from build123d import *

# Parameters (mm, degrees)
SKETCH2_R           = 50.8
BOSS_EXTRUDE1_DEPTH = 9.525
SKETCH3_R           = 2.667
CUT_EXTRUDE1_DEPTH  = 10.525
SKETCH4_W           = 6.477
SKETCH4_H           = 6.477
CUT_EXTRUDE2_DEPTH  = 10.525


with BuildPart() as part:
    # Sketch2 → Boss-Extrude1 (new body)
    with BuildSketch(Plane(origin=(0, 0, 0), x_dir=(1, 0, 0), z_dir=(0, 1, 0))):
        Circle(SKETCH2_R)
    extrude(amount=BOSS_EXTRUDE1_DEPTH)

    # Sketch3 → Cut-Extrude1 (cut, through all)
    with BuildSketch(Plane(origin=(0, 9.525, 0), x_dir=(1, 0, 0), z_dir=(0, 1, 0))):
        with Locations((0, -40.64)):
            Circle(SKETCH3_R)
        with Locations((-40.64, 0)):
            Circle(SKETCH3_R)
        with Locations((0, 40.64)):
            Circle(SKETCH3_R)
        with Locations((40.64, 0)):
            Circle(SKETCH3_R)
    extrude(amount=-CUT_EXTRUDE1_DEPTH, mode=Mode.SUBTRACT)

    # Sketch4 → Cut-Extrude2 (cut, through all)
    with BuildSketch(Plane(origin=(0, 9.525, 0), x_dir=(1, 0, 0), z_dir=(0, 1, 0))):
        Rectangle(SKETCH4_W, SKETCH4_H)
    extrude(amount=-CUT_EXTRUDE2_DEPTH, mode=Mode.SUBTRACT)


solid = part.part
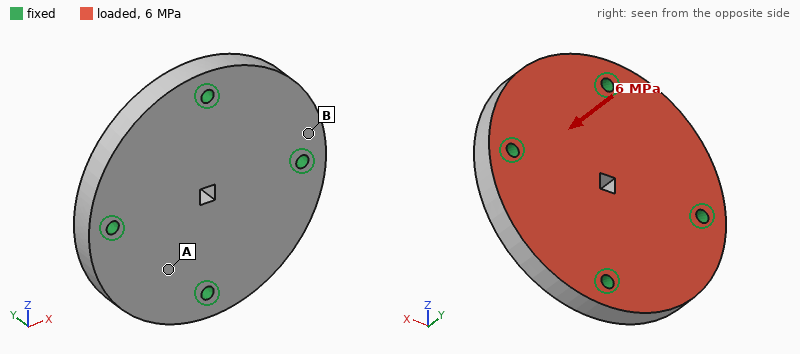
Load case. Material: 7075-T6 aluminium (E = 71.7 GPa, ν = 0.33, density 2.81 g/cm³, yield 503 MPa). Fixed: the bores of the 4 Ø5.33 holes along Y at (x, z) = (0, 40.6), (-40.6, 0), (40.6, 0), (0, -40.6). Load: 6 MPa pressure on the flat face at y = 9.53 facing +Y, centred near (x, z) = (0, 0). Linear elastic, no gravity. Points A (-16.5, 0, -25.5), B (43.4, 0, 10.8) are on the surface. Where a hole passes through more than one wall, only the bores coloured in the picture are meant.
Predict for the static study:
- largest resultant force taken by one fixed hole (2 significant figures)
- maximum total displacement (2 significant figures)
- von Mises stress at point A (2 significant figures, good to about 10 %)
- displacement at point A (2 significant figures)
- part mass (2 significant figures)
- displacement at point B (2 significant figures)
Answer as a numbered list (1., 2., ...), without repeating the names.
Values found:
1. 12 kN
2. 96 µm
3. 66 MPa
4. 60 µm
5. 210 g
6. 22 µm
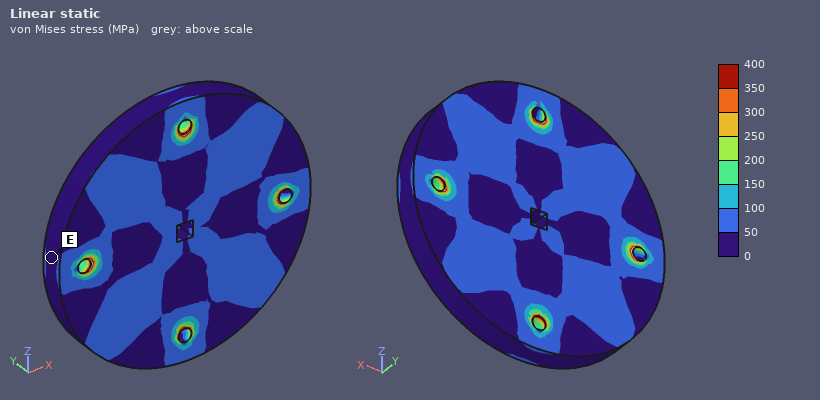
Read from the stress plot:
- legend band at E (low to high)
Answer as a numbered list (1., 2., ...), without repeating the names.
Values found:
1. 0 to 50 MPa
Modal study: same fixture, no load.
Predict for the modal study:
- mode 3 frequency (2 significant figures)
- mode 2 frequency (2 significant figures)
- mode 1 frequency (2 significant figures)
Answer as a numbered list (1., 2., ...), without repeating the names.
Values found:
1. 9900 Hz
2. 9200 Hz
3. 9200 Hz
